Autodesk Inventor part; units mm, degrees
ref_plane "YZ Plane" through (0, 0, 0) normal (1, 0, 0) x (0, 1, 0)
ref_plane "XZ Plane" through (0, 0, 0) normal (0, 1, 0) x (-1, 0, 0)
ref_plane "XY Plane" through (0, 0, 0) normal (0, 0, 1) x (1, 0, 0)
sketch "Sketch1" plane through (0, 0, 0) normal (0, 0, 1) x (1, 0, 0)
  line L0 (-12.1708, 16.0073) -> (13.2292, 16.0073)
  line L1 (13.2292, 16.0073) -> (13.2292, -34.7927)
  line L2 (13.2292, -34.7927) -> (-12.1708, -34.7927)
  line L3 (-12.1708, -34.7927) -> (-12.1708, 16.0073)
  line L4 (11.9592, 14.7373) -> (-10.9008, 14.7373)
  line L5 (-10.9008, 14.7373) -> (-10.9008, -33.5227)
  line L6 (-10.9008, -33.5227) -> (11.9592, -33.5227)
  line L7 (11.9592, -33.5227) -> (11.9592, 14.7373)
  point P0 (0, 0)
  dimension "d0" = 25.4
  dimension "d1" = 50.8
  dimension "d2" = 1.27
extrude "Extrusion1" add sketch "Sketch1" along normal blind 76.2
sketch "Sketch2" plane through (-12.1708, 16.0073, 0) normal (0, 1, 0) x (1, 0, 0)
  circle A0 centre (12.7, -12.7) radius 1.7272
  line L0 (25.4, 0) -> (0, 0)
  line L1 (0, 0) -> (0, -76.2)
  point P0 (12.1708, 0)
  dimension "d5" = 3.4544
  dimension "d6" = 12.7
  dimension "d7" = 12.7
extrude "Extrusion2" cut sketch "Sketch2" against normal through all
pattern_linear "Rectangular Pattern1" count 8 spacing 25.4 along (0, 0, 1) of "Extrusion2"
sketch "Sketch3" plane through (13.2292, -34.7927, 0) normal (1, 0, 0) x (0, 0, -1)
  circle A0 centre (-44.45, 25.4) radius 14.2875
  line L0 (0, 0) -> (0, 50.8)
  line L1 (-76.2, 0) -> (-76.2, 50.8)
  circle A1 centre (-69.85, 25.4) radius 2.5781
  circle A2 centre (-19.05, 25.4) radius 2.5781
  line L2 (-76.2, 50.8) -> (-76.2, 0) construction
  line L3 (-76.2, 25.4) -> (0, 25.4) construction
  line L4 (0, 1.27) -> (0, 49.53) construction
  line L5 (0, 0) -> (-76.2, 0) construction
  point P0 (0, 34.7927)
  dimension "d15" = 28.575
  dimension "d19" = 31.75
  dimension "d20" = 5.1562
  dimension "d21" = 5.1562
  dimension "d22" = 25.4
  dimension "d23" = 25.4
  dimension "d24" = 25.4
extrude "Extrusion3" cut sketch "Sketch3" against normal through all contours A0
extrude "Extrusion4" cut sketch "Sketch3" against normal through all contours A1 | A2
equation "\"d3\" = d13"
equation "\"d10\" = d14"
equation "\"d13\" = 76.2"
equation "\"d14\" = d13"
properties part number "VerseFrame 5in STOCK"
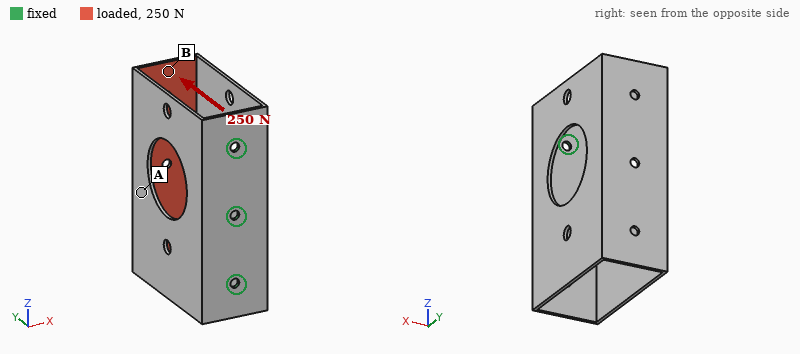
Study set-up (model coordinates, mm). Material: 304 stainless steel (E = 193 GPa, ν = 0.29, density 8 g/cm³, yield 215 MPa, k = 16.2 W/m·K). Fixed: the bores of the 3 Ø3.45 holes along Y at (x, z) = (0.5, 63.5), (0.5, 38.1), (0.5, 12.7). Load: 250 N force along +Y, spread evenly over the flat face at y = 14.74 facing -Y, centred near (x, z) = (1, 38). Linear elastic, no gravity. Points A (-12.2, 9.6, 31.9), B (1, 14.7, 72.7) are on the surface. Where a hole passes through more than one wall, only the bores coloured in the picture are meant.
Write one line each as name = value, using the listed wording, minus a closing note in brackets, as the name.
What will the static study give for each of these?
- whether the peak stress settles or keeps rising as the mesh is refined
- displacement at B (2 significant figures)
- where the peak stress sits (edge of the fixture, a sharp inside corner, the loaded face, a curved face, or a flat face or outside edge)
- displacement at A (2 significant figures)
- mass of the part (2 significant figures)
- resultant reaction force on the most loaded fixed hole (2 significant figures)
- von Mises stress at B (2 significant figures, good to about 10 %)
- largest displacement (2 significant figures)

whether the peak stress settles or keeps rising as the mesh is refined = keeps rising
displacement at B = 37 µm
where the peak stress sits = edge of the fixture
displacement at A = 22 µm
mass of the part = 100 g
resultant reaction force on the most loaded fixed hole = 85 N
von Mises stress at B = 34 MPa
largest displacement = 38 µm
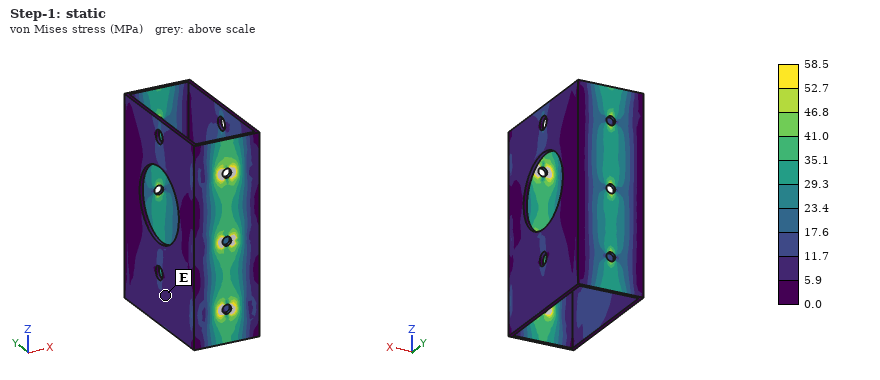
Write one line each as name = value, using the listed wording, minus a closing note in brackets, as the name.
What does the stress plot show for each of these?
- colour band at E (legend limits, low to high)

colour band at E = 5.9 to 11.7 MPa
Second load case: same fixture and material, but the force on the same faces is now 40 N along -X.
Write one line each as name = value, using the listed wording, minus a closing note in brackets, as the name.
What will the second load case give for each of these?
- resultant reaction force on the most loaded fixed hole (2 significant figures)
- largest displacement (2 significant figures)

resultant reaction force on the most loaded fixed hole = 16 N
largest displacement = 0.26 mm
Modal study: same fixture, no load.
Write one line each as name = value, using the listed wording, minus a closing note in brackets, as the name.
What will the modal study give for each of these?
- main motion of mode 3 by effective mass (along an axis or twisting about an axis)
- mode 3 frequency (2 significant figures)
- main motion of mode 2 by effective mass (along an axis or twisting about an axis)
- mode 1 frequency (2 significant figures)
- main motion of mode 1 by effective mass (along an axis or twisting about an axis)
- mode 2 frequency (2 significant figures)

main motion of mode 3 by effective mass = along Z
mode 3 frequency = 1100 Hz
main motion of mode 2 by effective mass = twisting about Y
mode 1 frequency = 300 Hz
main motion of mode 1 by effective mass = along X
mode 2 frequency = 1000 Hz
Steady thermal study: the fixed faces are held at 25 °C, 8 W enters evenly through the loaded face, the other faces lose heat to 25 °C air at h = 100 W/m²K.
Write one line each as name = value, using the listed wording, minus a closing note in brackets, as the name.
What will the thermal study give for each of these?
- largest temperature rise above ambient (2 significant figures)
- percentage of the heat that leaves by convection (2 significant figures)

largest temperature rise above ambient = 23 K
percentage of the heat that leaves by convection = 100 %
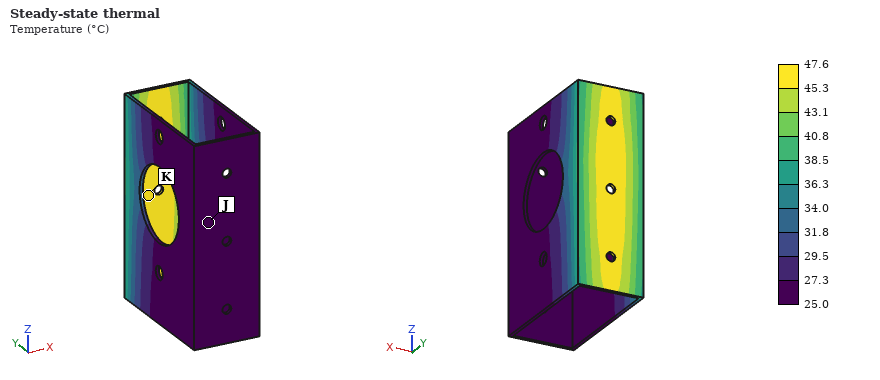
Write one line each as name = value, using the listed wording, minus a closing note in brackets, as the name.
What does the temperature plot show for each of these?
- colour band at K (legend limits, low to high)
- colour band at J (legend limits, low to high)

colour band at K = 45.3 to 47.6 °C
colour band at J = 25.0 to 27.3 °C
